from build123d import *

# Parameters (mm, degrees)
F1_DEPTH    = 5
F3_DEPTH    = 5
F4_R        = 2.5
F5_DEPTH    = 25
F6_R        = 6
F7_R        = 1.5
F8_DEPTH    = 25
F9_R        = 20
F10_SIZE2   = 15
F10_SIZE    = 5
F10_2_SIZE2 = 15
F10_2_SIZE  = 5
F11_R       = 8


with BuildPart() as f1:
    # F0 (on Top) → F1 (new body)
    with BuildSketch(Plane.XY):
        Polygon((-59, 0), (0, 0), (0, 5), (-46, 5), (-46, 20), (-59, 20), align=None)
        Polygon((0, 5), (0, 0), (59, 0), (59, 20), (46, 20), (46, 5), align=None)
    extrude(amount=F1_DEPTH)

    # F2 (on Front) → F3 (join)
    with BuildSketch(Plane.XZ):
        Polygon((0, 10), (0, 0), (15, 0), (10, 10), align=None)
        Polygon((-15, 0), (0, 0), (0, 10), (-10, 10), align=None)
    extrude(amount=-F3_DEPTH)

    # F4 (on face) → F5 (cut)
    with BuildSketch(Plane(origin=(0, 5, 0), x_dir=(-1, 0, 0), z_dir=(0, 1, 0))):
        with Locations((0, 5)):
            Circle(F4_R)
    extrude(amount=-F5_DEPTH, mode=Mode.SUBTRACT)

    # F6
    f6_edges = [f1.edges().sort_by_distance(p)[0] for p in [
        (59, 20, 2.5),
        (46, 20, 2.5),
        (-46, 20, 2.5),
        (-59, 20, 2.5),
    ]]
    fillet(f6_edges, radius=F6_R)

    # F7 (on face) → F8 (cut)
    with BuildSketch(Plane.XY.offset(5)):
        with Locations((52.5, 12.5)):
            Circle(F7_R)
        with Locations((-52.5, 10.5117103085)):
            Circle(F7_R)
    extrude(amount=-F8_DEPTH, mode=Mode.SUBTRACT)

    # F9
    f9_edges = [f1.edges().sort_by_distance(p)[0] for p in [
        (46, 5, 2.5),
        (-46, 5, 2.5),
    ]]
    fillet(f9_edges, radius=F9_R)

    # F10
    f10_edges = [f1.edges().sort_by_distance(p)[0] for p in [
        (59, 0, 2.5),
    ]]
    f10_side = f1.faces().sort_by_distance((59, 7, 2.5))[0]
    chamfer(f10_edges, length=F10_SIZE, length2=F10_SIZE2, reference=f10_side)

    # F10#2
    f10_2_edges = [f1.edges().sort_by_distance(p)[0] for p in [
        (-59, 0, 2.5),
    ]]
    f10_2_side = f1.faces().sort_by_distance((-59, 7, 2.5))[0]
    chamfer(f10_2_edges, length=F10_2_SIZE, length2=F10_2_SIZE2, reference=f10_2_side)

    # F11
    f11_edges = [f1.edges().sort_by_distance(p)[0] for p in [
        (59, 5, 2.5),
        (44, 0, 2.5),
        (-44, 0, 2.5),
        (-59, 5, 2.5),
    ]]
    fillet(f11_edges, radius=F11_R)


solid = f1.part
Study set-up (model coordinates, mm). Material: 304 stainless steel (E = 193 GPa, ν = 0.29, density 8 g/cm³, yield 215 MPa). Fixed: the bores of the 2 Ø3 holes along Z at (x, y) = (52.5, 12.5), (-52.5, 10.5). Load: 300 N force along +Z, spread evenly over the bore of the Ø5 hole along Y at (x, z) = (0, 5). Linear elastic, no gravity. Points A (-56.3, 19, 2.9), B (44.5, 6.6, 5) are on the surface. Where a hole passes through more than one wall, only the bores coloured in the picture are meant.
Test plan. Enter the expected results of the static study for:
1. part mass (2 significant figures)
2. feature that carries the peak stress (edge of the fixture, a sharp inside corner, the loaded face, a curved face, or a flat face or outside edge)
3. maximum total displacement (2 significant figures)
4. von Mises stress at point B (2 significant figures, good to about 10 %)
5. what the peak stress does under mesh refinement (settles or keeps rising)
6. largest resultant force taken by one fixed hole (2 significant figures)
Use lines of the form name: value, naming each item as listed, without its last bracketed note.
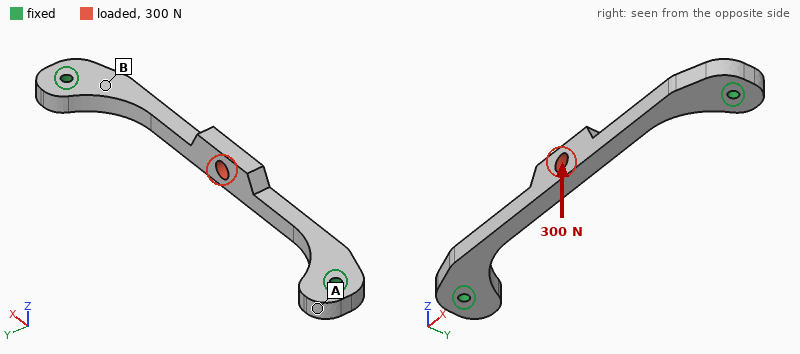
part mass: 42 g
feature that carries the peak stress: edge of the fixture
maximum total displacement: 86 µm
von Mises stress at point B: 58 MPa
what the peak stress does under mesh refinement: keeps rising
largest resultant force taken by one fixed hole: 160 N
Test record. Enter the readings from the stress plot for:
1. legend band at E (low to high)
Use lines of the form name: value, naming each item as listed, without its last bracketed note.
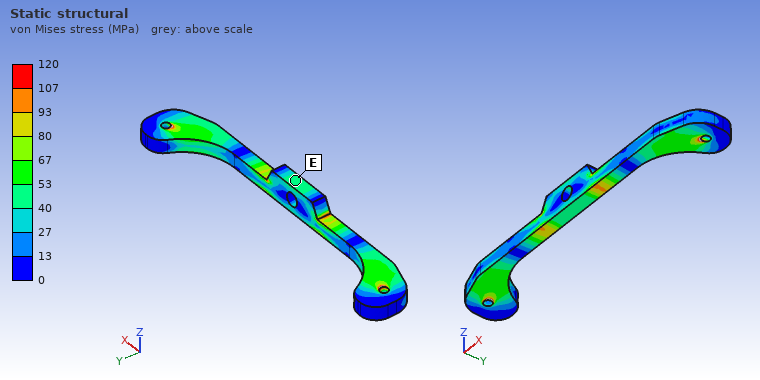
legend band at E: 40 to 53 MPa
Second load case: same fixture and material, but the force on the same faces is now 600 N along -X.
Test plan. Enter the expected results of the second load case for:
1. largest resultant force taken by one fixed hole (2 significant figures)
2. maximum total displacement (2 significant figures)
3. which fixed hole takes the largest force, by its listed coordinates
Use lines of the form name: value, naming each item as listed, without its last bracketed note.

largest resultant force taken by one fixed hole: 330 N
maximum total displacement: 9.4 µm
which fixed hole takes the largest force, by its listed coordinates: (-52.5, 10.5)
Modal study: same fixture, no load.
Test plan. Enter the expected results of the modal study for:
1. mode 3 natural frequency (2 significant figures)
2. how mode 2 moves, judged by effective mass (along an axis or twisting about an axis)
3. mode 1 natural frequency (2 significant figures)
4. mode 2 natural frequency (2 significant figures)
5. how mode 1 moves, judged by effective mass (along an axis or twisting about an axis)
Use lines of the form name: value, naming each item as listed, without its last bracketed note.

mode 3 natural frequency: 6300 Hz
how mode 2 moves, judged by effective mass: along Y
mode 1 natural frequency: 2600 Hz
mode 2 natural frequency: 3300 Hz
how mode 1 moves, judged by effective mass: along Z
